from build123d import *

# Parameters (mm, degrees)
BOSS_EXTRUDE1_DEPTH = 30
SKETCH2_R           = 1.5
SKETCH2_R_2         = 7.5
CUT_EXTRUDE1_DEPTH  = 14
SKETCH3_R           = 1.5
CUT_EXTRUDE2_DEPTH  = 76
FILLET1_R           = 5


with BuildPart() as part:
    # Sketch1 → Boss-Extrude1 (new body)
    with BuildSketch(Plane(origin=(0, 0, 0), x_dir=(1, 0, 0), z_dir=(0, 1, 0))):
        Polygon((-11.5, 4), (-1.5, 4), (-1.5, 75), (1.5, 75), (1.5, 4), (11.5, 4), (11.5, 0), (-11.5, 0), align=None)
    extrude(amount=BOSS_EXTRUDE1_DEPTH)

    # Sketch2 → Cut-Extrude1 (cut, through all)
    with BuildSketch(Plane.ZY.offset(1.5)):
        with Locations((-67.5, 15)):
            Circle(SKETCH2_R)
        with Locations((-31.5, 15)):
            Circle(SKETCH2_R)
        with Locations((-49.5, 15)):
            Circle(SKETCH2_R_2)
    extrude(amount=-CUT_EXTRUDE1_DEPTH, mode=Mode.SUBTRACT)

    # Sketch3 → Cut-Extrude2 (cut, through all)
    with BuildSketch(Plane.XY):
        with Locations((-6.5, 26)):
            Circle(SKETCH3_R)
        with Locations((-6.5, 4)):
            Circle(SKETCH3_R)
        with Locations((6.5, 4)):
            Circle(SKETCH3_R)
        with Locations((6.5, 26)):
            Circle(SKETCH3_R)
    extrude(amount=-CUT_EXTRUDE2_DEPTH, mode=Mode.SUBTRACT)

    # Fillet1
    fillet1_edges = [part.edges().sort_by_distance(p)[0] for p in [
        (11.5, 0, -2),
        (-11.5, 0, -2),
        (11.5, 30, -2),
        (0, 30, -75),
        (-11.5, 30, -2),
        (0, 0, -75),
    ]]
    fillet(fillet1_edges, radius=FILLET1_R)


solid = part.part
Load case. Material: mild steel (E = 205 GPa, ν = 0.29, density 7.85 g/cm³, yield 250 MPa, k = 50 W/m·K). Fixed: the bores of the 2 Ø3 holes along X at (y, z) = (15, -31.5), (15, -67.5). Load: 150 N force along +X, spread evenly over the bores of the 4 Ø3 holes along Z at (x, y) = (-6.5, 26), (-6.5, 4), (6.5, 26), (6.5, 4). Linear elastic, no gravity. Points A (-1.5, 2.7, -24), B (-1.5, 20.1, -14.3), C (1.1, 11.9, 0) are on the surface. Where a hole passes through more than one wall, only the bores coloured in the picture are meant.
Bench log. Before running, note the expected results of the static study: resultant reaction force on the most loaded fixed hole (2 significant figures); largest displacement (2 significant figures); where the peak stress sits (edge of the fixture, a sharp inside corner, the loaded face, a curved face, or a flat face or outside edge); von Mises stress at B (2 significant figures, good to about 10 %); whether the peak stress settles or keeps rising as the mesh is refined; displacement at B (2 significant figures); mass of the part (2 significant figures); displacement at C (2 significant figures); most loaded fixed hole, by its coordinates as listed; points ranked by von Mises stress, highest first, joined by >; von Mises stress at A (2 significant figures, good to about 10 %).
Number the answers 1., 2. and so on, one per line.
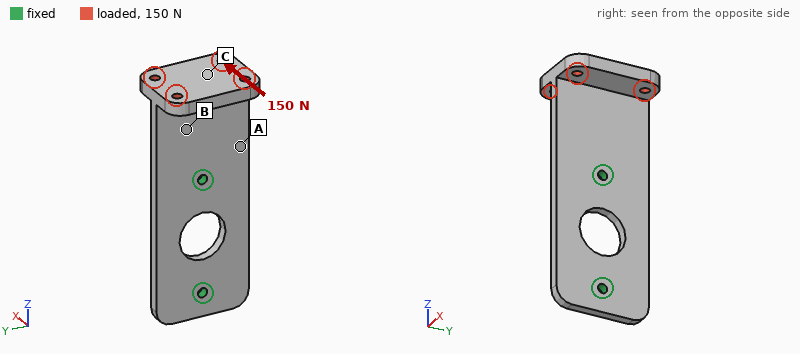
1. 190 N
2. 0.13 mm
3. edge of the fixture
4. 37 MPa
5. keeps rising
6. 0.048 mm
7. 66 g
8. 0.12 mm
9. (15, -31.5)
10. A > B > C
11. 65 MPa
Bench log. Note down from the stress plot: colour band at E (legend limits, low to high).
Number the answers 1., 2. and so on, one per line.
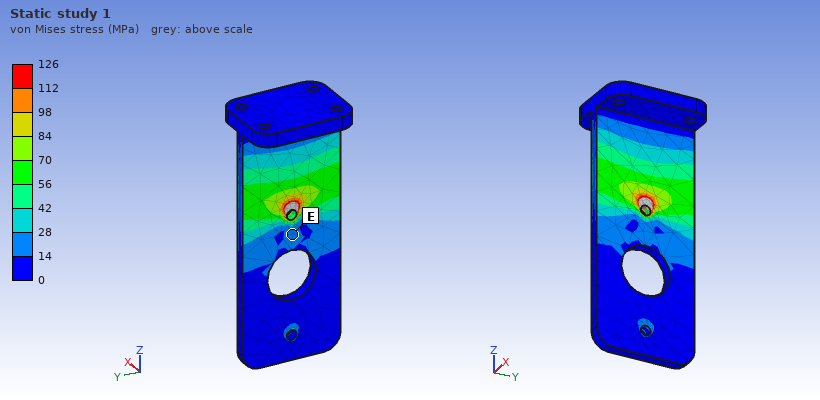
1. 14 to 28 MPa
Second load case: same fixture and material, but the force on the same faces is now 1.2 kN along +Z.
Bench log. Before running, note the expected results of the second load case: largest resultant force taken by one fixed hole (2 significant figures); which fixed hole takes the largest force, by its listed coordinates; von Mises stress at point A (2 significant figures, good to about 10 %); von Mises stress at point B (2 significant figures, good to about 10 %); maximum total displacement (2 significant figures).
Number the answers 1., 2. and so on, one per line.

1. 1.0 kN
2. (15, -31.5)
3. 9.6 MPa
4. 14 MPa
5. 6.5 µm
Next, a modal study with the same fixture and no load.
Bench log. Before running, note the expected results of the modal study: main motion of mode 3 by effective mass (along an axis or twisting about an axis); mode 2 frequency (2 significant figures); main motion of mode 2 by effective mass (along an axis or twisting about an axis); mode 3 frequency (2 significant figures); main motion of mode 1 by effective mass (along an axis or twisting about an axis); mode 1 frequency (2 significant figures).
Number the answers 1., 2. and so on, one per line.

1. along Y
2. 2600 Hz
3. twisting about Z
4. 5700 Hz
5. along X
6. 1200 Hz
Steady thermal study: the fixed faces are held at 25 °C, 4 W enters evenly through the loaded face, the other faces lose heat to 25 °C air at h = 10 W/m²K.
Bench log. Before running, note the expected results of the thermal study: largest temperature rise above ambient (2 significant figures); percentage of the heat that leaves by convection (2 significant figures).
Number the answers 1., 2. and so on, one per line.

1. 28 K
2. 18 %
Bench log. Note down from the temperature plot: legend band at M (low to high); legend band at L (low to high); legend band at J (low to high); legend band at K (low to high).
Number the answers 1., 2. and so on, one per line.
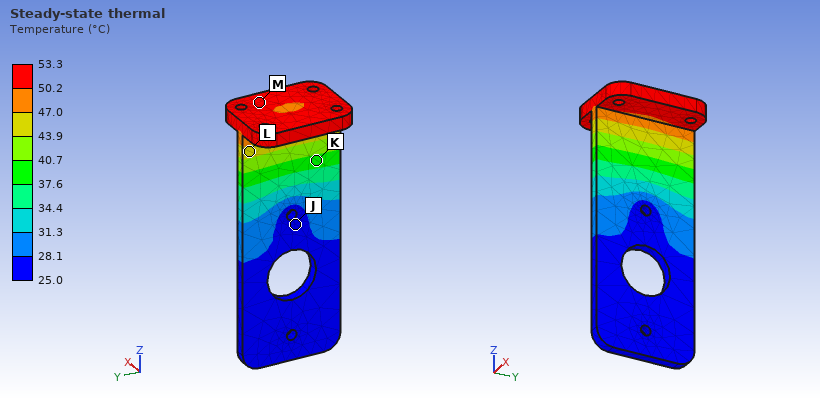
1. 50.2 to 53.3 °C
2. 43.9 to 47.0 °C
3. 25.0 to 28.1 °C
4. 37.6 to 40.7 °C
